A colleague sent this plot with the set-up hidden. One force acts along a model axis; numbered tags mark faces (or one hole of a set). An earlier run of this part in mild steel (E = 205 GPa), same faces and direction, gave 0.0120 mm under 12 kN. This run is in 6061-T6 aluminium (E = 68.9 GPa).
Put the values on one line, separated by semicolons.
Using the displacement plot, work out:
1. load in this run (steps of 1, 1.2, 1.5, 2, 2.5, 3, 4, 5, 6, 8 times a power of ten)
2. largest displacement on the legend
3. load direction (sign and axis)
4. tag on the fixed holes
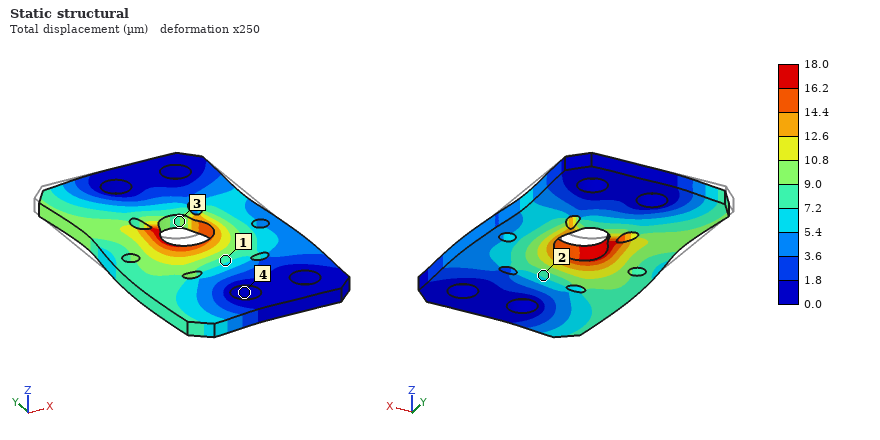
6 kN; 18.0 µm; -Y; 4
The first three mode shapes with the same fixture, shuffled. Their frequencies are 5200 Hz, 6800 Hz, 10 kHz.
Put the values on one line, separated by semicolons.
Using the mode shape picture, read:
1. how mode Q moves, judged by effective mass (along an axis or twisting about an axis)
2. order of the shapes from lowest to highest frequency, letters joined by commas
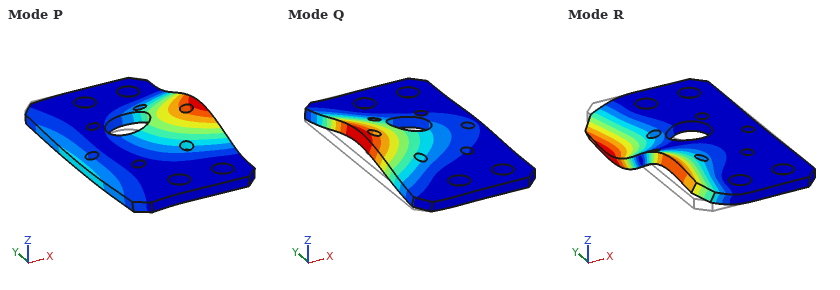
along Z; Q, P, R
